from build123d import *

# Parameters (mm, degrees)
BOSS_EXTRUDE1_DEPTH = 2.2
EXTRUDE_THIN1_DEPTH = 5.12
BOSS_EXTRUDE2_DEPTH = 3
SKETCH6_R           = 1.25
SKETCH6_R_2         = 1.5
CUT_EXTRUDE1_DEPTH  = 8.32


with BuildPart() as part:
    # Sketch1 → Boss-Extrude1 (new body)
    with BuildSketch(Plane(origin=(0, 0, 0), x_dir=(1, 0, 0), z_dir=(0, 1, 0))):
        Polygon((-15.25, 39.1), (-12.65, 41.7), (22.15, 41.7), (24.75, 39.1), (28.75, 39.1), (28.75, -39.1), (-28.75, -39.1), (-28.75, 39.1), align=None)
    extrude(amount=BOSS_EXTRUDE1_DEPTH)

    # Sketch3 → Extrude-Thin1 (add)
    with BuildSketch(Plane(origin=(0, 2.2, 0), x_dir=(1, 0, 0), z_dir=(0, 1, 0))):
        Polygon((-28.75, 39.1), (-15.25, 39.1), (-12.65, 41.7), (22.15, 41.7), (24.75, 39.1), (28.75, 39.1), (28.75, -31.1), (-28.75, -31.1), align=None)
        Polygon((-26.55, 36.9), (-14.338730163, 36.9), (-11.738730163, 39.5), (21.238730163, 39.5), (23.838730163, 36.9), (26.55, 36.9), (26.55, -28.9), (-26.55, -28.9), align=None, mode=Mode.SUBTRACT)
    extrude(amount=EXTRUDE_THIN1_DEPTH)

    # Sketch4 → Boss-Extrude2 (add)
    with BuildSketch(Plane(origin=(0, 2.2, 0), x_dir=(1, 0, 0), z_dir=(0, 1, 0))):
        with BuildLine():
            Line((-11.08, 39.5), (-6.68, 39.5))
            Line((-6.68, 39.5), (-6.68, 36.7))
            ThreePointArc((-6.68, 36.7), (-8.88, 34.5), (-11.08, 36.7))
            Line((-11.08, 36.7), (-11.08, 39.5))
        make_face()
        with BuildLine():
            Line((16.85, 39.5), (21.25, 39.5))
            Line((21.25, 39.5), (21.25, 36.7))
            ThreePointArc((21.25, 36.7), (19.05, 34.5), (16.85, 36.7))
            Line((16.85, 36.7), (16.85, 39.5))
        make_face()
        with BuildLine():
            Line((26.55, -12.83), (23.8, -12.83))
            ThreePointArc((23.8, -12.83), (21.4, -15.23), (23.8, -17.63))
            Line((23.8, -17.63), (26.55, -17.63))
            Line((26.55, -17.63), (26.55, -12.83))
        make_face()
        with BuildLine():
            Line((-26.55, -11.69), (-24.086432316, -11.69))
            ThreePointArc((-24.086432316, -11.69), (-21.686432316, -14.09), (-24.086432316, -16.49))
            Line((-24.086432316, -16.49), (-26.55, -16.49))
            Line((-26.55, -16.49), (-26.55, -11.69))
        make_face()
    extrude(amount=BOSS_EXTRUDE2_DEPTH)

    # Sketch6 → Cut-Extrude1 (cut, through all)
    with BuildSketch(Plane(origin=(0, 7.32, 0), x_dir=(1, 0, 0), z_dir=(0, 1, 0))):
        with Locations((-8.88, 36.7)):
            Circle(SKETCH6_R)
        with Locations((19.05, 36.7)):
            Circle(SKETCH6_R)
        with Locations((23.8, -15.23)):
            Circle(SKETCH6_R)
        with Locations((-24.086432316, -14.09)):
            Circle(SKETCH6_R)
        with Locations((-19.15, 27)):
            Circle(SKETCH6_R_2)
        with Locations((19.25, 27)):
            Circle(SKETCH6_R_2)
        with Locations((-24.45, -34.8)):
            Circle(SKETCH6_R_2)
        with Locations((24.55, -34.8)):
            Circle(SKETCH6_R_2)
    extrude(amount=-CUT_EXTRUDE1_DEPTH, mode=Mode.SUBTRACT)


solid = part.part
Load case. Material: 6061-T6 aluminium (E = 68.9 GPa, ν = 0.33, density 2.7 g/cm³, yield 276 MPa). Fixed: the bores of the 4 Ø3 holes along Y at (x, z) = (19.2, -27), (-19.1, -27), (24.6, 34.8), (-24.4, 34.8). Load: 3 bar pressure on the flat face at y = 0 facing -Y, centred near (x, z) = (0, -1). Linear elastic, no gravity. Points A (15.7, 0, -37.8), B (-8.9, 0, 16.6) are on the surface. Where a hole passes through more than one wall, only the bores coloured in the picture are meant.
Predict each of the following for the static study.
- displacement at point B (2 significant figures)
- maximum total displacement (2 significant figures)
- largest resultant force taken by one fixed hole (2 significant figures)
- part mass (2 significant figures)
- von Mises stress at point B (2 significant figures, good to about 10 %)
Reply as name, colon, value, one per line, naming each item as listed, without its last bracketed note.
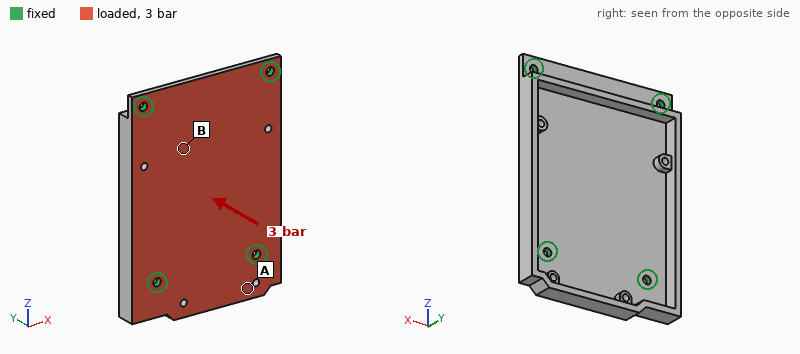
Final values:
displacement at point B: 0.12 mm
maximum total displacement: 0.16 mm
largest resultant force taken by one fixed hole: 430 N
part mass: 35 g
von Mises stress at point B: 33 MPa
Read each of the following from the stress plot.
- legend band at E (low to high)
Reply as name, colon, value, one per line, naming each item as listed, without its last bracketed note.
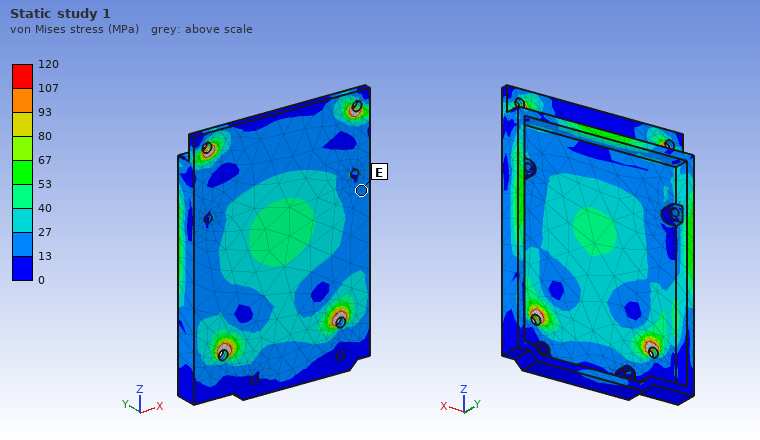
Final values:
legend band at E: 13 to 27 MPa
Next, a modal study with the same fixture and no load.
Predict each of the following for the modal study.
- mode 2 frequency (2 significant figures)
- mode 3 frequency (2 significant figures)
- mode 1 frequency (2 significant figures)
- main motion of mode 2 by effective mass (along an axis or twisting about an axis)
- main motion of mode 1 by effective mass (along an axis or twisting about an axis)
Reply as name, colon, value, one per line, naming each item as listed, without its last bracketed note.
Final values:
mode 2 frequency: 5100 Hz
mode 3 frequency: 5700 Hz
mode 1 frequency: 3300 Hz
main motion of mode 2 by effective mass: twisting about Z
main motion of mode 1 by effective mass: along Y
